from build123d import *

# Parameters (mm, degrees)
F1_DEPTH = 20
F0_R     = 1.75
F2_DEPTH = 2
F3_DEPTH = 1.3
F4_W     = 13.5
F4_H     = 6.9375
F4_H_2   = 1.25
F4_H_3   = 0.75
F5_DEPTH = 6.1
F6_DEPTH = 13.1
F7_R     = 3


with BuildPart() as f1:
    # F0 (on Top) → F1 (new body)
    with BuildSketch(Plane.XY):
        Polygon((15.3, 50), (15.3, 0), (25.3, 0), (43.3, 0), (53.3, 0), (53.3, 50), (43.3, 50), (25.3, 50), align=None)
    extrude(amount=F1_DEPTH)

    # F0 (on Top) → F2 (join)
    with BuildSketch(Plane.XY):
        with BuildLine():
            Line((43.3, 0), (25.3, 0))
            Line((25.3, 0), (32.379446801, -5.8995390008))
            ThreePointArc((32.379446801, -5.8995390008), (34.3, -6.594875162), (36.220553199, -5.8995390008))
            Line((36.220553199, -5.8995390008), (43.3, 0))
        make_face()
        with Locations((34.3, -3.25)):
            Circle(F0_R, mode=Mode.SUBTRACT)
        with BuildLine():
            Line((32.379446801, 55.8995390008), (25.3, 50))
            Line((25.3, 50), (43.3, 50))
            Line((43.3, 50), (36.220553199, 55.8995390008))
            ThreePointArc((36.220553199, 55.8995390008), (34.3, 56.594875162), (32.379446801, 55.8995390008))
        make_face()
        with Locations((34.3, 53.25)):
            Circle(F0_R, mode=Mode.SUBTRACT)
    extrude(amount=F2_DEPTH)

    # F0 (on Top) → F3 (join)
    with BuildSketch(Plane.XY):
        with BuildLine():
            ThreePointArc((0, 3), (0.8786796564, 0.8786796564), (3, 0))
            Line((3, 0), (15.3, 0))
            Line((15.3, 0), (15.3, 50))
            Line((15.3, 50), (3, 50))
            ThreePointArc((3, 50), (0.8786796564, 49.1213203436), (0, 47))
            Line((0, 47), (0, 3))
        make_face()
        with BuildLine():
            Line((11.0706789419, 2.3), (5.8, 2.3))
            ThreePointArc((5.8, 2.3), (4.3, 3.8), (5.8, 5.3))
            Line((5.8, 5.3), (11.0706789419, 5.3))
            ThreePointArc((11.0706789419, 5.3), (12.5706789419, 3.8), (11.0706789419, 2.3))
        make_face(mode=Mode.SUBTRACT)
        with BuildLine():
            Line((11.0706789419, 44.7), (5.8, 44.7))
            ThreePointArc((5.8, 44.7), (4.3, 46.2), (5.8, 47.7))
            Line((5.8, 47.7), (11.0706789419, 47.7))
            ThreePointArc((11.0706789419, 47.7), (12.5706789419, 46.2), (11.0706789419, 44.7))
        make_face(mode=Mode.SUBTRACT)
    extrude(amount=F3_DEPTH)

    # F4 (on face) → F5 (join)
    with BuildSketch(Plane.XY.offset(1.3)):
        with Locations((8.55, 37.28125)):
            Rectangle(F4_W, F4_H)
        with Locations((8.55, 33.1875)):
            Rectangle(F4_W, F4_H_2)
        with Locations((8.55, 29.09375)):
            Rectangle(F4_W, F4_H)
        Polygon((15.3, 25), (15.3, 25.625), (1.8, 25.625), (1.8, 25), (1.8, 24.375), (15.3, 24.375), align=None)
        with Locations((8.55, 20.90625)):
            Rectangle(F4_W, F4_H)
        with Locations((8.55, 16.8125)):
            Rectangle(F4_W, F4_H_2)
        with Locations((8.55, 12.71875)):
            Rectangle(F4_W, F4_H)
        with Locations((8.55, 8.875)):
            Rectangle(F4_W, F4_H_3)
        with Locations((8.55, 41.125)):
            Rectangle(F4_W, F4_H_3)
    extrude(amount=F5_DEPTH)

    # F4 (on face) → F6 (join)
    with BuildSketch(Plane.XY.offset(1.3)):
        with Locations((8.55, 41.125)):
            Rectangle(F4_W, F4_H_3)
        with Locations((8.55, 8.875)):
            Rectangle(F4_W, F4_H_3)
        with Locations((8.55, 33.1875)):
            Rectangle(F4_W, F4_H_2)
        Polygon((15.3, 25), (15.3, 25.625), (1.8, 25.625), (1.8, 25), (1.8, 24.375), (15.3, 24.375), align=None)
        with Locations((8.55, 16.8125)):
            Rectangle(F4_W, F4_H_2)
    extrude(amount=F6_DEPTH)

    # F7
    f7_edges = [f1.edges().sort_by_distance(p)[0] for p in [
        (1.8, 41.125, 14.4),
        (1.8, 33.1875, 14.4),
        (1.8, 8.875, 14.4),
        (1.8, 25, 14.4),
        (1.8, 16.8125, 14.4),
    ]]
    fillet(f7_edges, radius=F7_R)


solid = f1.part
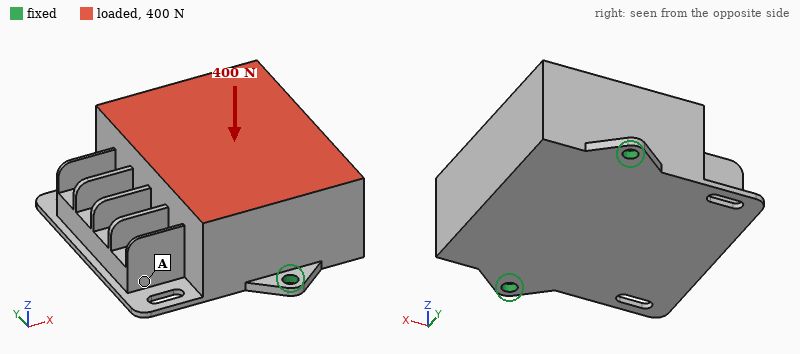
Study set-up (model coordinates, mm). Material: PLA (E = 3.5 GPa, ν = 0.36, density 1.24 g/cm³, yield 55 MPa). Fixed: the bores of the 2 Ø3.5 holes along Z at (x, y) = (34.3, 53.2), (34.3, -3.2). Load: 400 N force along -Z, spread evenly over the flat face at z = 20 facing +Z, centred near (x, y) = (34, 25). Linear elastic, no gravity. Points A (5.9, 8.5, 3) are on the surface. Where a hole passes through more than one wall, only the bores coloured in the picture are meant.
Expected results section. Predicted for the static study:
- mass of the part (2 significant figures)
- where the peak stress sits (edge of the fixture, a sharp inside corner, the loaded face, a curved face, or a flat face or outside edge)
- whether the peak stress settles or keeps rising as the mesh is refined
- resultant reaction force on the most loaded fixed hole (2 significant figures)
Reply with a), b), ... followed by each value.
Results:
a) 53 g
b) edge of the fixture
c) keeps rising
d) 230 N
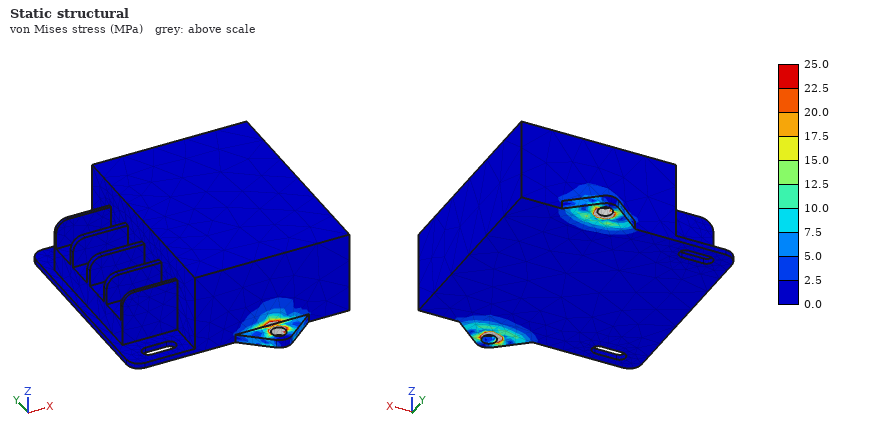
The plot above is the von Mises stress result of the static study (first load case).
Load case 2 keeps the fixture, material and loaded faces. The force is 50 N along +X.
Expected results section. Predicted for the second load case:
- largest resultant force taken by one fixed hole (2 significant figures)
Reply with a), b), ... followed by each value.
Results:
a) 25 N
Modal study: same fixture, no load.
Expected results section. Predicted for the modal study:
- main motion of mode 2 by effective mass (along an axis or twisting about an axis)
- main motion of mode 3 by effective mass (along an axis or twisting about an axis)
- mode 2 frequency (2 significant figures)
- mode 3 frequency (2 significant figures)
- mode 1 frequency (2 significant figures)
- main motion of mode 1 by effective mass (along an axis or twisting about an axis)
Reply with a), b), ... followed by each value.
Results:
a) along Z
b) along Y
c) 1700 Hz
d) 2500 Hz
e) 270 Hz
f) along X
